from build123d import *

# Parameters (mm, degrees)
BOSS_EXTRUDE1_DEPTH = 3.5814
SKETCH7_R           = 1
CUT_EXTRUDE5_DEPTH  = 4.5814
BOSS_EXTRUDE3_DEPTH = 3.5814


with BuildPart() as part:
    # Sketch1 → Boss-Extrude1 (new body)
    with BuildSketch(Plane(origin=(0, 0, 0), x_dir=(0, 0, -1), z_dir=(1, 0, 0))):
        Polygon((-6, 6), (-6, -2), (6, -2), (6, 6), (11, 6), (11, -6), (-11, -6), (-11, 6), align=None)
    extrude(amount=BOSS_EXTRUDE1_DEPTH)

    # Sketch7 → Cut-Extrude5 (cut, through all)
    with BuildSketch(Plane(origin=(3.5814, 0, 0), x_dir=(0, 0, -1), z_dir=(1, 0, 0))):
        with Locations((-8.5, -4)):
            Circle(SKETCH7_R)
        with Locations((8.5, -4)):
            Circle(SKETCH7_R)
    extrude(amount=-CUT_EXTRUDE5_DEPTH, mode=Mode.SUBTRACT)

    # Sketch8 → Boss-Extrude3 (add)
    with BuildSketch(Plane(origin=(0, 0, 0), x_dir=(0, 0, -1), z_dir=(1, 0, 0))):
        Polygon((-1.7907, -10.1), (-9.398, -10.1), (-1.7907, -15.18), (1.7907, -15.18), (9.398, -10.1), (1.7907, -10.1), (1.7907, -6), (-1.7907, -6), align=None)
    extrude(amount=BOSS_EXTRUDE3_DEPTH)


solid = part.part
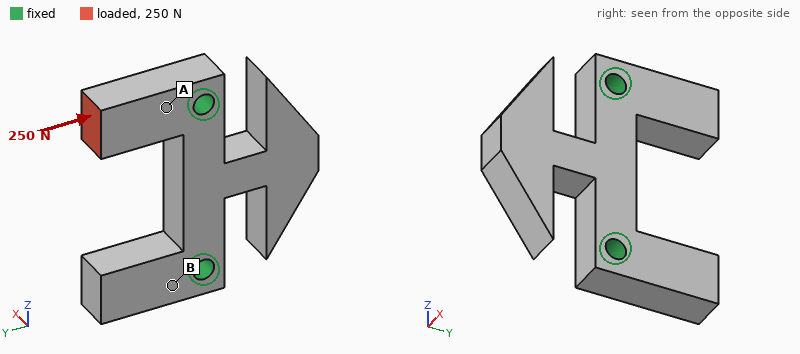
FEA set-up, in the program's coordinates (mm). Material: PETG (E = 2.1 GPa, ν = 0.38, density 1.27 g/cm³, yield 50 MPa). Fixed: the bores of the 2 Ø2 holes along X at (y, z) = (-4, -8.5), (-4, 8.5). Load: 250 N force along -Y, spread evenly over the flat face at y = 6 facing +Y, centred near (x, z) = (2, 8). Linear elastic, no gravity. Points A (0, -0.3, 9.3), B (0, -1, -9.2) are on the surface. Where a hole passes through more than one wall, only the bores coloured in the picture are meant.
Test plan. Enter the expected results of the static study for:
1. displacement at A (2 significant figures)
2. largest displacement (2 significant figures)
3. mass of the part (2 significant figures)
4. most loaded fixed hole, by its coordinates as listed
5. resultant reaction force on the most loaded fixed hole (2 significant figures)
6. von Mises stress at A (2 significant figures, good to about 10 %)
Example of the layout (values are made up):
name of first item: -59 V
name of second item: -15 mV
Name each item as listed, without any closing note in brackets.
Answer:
displacement at A: 25 µm
largest displacement: 71 µm
mass of the part: 1.1 g
most loaded fixed hole, by its coordinates as listed: (-4, 8.5)
resultant reaction force on the most loaded fixed hole: 250 N
von Mises stress at A: 15 MPa
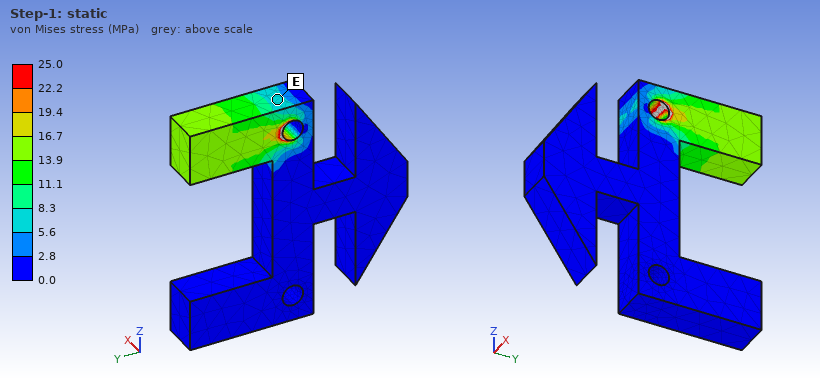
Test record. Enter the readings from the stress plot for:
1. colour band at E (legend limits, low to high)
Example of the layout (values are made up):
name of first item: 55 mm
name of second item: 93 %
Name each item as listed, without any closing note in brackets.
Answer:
colour band at E: 5.6 to 8.3 MPa
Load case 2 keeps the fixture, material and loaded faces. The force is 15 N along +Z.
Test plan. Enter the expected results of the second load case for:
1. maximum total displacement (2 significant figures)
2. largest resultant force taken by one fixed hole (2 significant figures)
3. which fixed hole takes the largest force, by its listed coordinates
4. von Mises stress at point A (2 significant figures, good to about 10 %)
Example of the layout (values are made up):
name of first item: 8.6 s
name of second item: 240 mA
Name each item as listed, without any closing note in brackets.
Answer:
maximum total displacement: 92 µm
largest resultant force taken by one fixed hole: 13 N
which fixed hole takes the largest force, by its listed coordinates: (-4, 8.5)
von Mises stress at point A: 2.8 MPa
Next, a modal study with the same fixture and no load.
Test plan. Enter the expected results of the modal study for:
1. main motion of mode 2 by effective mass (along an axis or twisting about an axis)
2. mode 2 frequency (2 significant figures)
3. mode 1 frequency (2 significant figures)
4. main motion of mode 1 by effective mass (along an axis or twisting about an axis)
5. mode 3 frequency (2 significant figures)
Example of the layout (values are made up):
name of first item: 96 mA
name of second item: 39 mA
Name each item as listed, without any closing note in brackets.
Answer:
main motion of mode 2 by effective mass: along Z
mode 2 frequency: 3200 Hz
mode 1 frequency: 2400 Hz
main motion of mode 1 by effective mass: along X
mode 3 frequency: 4200 Hz
